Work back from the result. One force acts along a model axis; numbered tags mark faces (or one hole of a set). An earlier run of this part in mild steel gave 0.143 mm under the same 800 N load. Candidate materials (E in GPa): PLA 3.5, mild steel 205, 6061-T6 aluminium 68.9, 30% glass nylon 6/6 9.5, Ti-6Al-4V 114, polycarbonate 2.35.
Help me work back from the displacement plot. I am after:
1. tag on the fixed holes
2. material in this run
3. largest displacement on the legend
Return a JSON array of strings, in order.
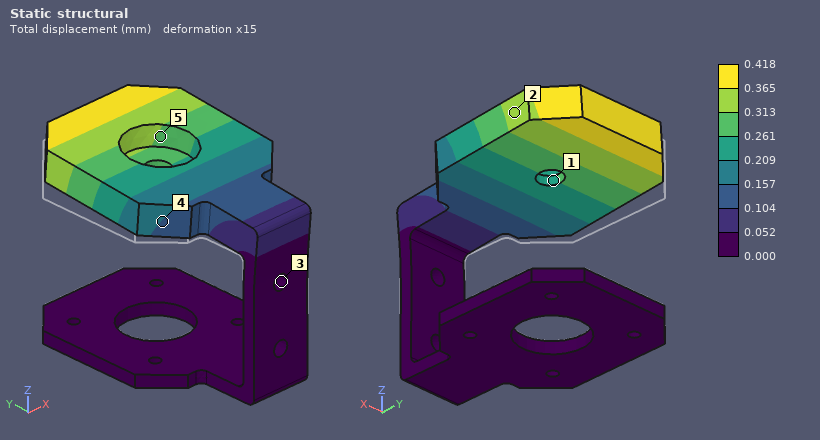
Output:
["3", "6061-T6 aluminium", "0.418 mm"]
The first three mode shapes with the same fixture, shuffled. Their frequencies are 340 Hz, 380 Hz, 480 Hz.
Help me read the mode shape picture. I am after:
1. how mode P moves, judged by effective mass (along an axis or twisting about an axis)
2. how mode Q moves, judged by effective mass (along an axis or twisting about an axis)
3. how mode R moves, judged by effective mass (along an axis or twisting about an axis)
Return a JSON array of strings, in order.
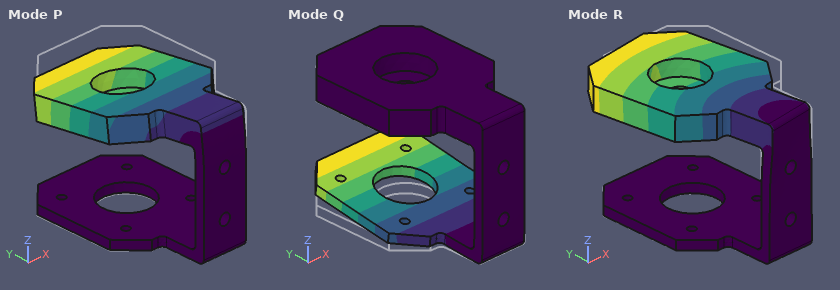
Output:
["along Z", "along Z", "along X"]
